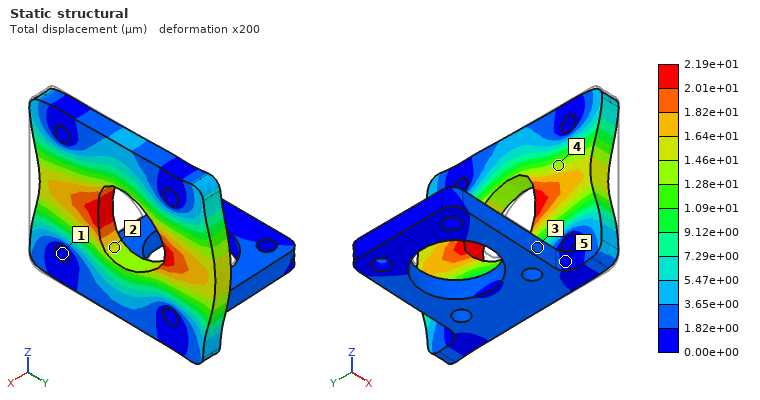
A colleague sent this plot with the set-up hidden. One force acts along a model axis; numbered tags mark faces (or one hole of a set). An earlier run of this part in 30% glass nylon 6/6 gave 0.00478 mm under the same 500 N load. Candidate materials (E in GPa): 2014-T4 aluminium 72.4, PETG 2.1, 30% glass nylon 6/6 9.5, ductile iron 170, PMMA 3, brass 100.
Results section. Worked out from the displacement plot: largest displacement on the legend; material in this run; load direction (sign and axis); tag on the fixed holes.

2.19e+01 µm
PETG
+Y
1
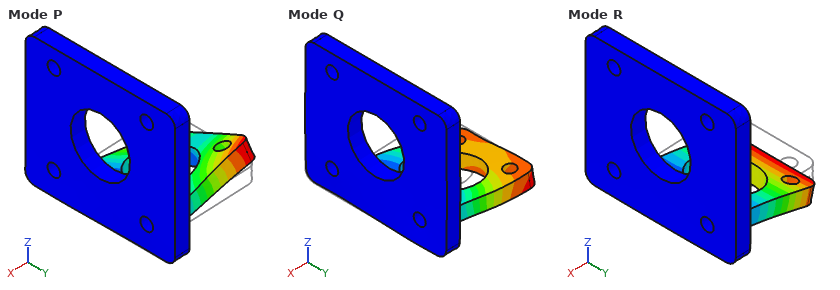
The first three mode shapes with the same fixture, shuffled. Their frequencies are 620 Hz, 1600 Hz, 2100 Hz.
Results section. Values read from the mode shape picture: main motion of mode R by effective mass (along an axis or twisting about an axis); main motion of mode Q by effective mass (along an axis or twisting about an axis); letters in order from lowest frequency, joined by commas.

along Z
along Y
R, P, Q
